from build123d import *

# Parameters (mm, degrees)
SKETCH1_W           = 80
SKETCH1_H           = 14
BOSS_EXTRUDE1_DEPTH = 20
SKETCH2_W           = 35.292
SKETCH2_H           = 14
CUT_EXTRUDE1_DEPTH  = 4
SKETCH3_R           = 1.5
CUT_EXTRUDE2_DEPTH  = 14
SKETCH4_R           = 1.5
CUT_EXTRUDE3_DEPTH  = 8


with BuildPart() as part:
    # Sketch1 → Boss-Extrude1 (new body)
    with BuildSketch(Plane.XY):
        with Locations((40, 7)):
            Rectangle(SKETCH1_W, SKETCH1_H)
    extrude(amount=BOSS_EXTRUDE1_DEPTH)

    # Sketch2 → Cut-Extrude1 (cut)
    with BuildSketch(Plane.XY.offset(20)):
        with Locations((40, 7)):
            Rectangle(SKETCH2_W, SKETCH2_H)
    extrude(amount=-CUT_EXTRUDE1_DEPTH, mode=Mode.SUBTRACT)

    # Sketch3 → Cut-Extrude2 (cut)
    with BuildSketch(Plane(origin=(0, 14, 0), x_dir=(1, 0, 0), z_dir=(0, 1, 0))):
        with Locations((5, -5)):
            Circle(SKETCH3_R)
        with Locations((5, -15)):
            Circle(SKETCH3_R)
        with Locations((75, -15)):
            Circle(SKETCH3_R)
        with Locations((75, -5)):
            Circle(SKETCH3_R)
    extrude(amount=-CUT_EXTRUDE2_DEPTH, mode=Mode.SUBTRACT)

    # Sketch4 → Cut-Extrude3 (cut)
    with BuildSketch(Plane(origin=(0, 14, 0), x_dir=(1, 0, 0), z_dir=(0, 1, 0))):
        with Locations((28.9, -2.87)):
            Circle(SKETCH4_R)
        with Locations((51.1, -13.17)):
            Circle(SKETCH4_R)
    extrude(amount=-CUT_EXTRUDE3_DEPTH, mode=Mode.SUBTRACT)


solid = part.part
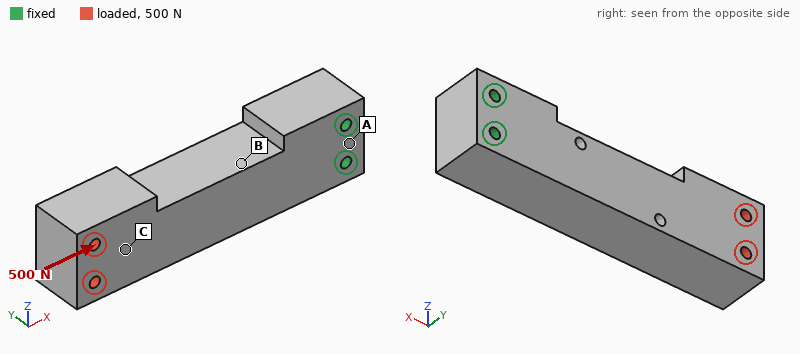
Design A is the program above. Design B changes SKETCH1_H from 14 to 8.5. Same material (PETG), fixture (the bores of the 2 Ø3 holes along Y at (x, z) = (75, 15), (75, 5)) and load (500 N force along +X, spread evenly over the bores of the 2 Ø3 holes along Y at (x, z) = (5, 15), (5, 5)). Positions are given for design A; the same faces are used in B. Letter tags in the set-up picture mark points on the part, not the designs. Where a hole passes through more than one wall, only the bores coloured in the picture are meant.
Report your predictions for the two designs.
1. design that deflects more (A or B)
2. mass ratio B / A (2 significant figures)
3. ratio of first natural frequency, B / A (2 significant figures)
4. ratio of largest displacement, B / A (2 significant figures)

B
0.61
0.62
1.7
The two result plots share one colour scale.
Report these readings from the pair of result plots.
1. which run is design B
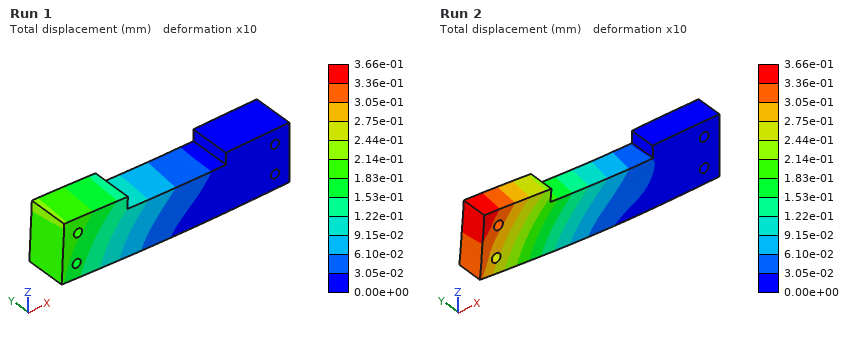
Run 2
